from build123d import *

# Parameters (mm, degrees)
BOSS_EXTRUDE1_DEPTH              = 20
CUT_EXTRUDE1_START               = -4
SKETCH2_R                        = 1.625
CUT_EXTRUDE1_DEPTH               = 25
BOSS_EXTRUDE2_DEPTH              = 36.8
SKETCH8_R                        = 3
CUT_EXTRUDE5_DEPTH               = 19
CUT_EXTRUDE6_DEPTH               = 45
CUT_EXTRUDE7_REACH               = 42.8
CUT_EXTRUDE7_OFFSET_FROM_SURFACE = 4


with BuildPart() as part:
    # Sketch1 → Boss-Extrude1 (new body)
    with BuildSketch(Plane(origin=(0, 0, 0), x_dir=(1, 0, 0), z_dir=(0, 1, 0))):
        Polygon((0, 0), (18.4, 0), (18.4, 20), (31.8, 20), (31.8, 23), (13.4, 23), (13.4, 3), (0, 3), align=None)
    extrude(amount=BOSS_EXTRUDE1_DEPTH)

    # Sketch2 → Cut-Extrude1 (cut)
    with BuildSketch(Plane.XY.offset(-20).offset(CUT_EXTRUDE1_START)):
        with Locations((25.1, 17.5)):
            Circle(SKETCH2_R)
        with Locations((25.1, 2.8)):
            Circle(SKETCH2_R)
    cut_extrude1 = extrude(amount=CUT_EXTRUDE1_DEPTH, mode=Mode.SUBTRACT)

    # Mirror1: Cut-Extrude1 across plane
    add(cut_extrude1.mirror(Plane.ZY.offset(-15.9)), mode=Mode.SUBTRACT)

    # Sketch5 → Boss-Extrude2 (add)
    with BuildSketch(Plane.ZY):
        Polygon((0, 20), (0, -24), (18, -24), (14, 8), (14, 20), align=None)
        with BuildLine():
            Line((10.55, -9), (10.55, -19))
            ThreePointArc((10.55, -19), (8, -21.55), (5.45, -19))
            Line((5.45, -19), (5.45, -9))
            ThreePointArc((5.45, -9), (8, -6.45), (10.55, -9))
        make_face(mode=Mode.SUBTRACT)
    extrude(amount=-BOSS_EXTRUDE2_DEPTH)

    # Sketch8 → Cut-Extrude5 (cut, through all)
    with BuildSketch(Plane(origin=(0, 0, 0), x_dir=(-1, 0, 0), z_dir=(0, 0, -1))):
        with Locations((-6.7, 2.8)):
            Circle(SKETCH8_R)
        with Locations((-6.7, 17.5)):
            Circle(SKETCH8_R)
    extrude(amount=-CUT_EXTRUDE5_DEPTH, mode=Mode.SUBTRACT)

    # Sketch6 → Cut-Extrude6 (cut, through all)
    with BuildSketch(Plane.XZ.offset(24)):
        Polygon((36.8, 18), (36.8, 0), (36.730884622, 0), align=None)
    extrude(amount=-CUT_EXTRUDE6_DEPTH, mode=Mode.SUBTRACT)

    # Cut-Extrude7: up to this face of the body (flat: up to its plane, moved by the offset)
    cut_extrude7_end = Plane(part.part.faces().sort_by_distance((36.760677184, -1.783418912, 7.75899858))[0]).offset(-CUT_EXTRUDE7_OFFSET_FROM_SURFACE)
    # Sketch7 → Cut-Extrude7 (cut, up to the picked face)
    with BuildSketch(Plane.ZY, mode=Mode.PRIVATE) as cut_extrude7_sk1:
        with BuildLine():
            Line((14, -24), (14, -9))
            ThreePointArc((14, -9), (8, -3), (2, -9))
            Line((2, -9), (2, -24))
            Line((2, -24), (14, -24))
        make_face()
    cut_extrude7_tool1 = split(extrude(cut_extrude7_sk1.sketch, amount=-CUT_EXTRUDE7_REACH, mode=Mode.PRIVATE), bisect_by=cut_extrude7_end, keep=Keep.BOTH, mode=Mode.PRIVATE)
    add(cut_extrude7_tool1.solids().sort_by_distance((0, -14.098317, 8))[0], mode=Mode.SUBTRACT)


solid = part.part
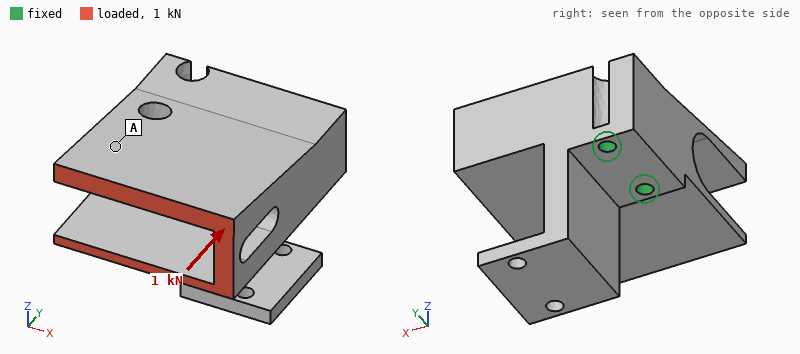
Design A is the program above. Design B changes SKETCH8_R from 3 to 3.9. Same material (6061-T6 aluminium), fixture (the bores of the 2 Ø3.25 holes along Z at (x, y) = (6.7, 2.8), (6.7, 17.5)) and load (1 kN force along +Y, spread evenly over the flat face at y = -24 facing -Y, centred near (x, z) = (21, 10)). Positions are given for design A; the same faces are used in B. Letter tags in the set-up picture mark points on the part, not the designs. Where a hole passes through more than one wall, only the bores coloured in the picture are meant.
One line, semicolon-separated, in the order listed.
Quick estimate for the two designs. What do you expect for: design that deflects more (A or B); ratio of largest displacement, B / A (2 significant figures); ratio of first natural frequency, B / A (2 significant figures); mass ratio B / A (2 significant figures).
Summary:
B; 1.2; 0.95; 0.98
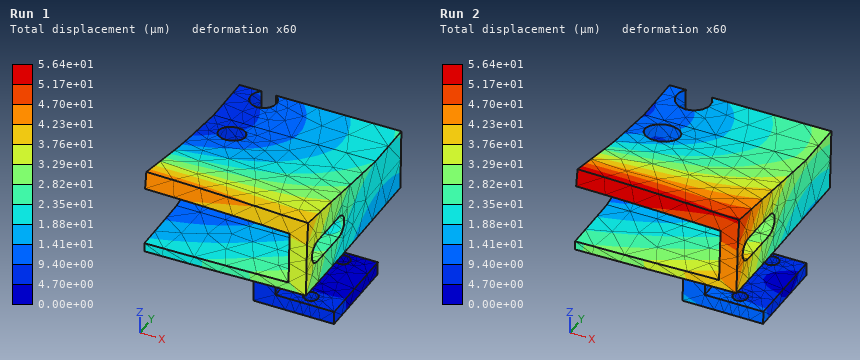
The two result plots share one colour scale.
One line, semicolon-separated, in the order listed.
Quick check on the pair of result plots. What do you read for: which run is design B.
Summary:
Run 2
